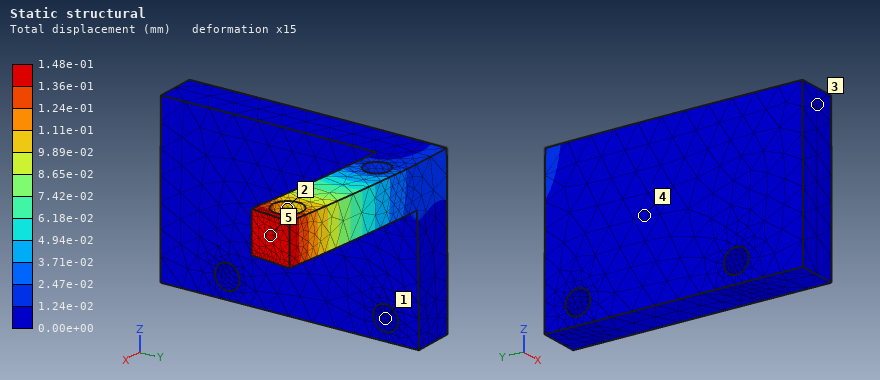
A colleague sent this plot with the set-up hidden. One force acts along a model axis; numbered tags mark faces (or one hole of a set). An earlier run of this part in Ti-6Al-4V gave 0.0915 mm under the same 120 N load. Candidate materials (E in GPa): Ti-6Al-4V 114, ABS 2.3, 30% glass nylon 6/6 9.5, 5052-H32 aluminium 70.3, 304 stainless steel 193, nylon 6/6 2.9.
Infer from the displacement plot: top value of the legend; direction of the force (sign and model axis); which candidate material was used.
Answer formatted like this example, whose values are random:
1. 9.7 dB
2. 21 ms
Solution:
1. 1.48e-01 mm
2. -Y
3. 5052-H32 aluminium
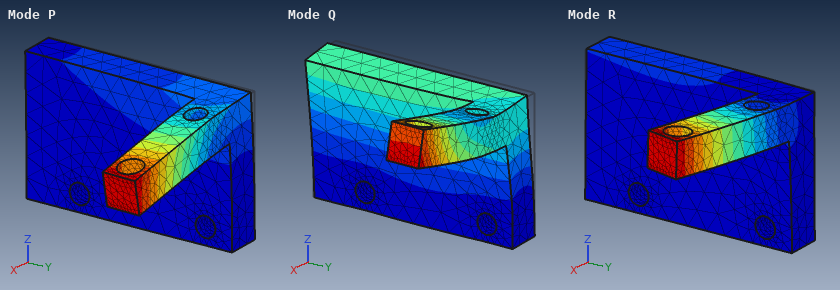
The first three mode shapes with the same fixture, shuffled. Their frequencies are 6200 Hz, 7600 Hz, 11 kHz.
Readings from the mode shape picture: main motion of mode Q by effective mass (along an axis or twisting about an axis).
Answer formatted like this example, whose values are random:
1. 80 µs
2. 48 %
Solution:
1. along X
